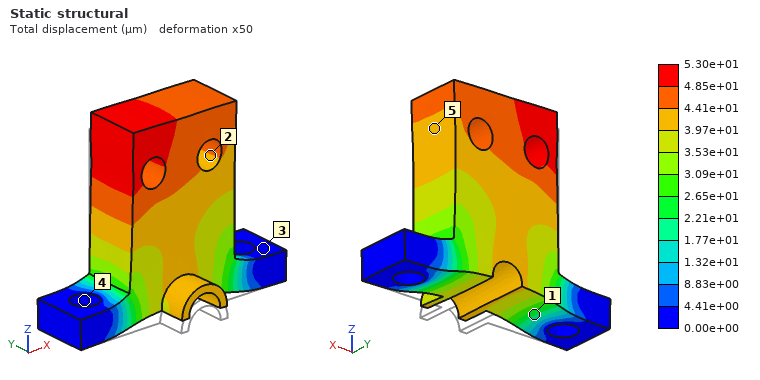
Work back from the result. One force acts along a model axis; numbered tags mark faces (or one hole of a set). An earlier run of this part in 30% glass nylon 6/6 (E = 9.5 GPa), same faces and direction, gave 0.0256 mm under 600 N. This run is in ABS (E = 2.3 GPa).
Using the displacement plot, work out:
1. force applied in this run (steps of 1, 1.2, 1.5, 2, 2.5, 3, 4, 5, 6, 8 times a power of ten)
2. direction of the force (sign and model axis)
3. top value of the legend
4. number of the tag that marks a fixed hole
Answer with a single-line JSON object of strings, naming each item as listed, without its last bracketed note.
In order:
{"force applied in this run": "300 N", "direction of the force": "+Z", "top value of the legend": "5.30e+01 µm", "number of the tag that marks a fixed hole": "4"}
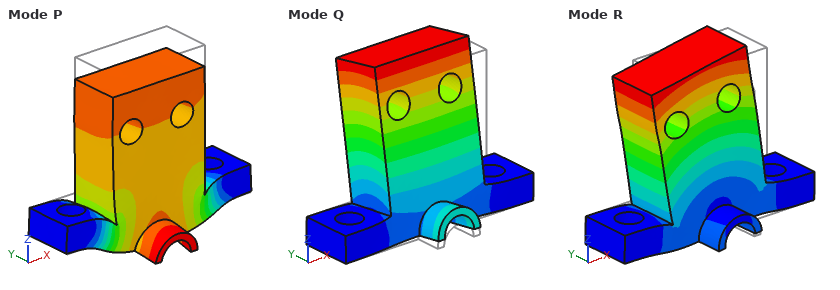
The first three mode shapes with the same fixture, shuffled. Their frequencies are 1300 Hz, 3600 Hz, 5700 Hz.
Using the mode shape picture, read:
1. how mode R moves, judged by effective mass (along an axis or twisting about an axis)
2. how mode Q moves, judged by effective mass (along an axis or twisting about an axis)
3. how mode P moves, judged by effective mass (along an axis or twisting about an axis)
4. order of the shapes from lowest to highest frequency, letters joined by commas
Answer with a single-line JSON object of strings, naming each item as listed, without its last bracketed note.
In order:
{"how mode R moves, judged by effective mass": "along X", "how mode Q moves, judged by effective mass": "along Y", "how mode P moves, judged by effective mass": "along Z", "order of the shapes from lowest to highest frequency, letters joined by commas": "Q, R, P"}
